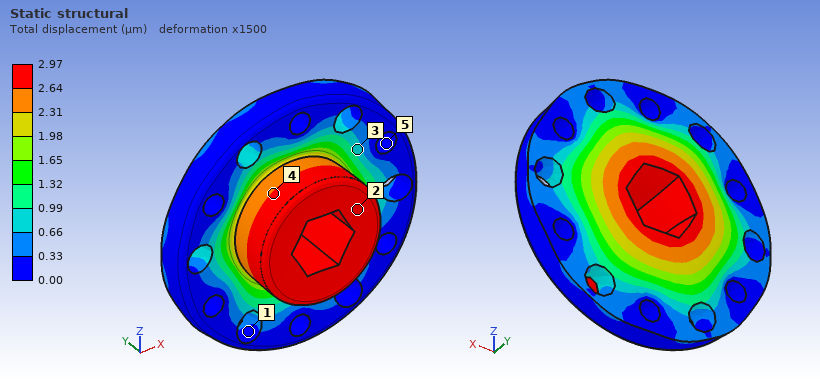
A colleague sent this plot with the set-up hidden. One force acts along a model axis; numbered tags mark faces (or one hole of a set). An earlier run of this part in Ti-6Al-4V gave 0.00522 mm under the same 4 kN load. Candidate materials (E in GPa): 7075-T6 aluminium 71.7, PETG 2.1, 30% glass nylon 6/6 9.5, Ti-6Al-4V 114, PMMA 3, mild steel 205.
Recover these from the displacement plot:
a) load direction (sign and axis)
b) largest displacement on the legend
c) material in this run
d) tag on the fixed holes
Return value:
+Y
2.97 µm
mild steel
5
